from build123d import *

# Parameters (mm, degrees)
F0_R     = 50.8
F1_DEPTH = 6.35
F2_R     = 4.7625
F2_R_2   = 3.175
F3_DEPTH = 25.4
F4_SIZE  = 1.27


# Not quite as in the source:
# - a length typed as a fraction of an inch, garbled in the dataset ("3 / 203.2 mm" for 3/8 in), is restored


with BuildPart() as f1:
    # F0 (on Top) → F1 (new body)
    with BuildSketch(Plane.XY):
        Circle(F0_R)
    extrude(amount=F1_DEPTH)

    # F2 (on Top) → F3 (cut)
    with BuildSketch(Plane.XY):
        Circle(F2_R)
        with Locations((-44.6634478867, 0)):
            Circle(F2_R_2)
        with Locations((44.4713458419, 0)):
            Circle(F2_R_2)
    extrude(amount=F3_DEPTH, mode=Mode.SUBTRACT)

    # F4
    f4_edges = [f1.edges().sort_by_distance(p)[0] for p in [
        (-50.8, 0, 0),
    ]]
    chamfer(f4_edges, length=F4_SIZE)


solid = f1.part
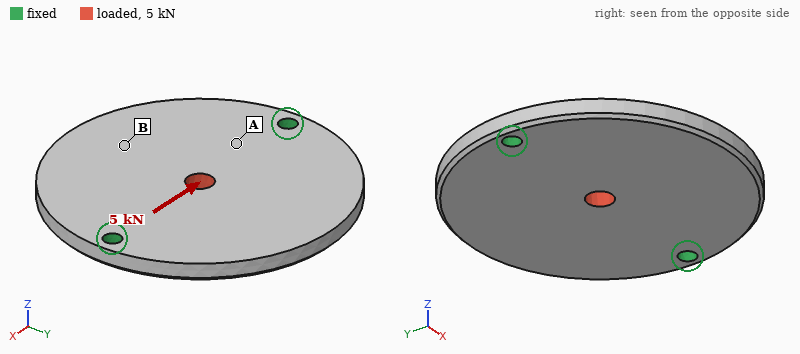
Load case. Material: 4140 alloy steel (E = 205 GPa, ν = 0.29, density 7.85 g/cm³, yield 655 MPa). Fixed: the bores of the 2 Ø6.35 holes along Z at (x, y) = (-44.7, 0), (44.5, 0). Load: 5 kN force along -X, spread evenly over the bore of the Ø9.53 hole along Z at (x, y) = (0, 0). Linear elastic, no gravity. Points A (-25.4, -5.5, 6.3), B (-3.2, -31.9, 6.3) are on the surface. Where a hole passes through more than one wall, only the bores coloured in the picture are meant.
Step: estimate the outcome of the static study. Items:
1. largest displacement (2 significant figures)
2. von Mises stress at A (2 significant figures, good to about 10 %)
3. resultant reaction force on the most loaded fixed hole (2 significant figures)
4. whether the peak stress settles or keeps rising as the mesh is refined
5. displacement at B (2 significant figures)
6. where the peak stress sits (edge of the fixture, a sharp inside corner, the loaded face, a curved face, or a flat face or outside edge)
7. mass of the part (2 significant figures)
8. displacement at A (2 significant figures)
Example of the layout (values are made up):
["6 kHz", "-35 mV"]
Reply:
["3.7 µm", "15 MPa", "2.5 kN", "keeps rising", "1.8 µm", "edge of the fixture", "400 g", "1.7 µm"]
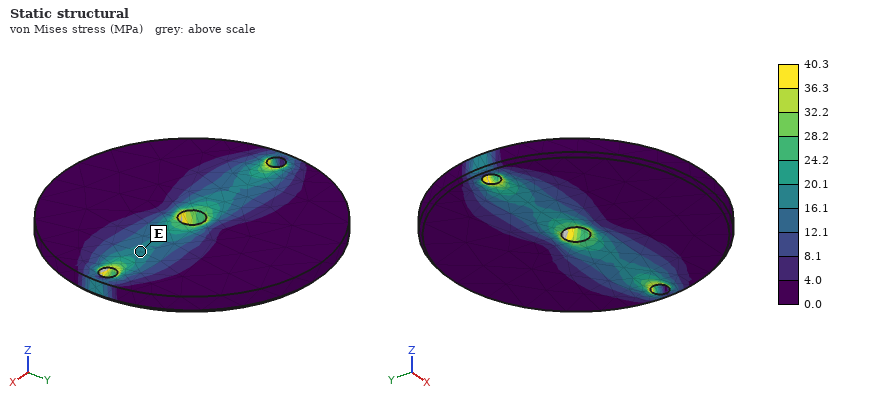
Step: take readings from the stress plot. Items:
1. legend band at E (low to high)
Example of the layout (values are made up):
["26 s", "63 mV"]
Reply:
["16.1 to 20.1 MPa"]
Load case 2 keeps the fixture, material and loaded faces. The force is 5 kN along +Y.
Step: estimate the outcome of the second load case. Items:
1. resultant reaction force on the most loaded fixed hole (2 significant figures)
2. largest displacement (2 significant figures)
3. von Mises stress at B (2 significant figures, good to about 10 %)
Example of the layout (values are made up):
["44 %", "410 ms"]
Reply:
["2.5 kN", "5.1 µm", "8.7 MPa"]
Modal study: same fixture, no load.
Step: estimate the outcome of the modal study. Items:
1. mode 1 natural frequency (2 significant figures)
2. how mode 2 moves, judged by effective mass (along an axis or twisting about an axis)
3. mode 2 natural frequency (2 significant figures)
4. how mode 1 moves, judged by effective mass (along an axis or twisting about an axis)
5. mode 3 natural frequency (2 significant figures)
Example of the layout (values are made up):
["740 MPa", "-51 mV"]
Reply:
["1600 Hz", "along Z", "2100 Hz", "twisting about X", "4900 Hz"]
